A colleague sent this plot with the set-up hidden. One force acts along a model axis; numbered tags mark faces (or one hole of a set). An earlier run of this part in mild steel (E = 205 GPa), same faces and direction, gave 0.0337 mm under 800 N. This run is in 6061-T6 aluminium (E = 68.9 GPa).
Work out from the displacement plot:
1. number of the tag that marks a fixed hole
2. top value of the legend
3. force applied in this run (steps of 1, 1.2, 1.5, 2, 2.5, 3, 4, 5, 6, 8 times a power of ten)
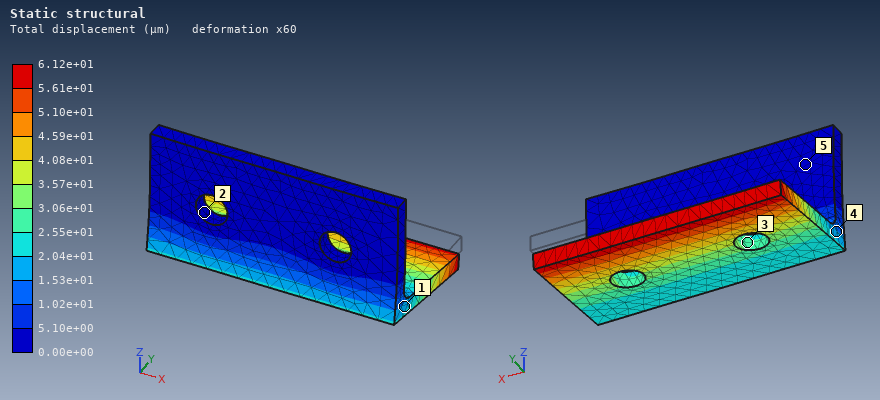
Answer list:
2
6.12e+01 µm
500 N
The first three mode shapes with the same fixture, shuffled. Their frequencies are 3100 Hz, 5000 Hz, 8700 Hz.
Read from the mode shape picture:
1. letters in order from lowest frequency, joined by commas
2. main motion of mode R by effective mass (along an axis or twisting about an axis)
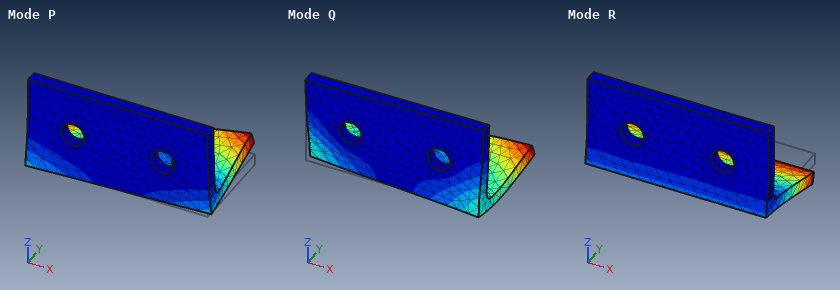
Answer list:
R, P, Q
along Z
